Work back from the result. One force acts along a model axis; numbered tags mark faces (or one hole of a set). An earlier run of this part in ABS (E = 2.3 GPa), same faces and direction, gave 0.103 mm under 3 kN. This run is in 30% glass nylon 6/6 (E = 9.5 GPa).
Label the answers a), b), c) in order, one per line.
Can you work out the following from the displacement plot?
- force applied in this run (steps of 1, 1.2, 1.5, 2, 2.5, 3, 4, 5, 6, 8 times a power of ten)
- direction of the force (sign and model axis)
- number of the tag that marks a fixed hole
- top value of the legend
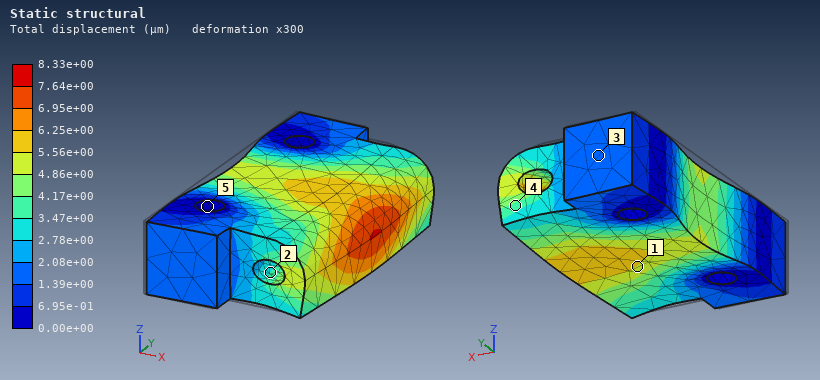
a) 1 kN
b) +X
c) 5
d) 8.33e+00 µm
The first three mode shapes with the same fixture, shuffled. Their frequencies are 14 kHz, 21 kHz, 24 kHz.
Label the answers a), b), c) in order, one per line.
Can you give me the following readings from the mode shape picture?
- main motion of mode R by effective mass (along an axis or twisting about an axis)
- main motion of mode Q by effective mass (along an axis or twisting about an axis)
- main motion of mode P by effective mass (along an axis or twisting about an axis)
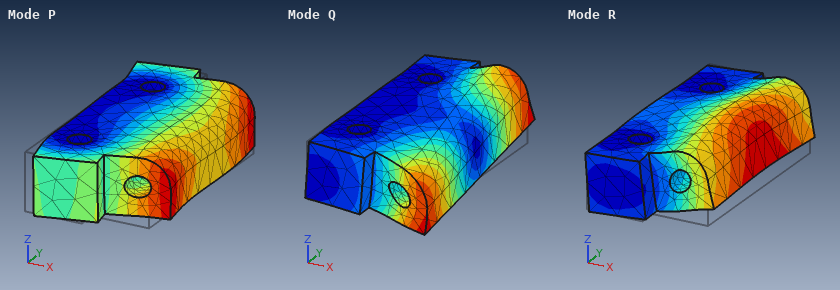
a) along Z
b) twisting about X
c) along Y
